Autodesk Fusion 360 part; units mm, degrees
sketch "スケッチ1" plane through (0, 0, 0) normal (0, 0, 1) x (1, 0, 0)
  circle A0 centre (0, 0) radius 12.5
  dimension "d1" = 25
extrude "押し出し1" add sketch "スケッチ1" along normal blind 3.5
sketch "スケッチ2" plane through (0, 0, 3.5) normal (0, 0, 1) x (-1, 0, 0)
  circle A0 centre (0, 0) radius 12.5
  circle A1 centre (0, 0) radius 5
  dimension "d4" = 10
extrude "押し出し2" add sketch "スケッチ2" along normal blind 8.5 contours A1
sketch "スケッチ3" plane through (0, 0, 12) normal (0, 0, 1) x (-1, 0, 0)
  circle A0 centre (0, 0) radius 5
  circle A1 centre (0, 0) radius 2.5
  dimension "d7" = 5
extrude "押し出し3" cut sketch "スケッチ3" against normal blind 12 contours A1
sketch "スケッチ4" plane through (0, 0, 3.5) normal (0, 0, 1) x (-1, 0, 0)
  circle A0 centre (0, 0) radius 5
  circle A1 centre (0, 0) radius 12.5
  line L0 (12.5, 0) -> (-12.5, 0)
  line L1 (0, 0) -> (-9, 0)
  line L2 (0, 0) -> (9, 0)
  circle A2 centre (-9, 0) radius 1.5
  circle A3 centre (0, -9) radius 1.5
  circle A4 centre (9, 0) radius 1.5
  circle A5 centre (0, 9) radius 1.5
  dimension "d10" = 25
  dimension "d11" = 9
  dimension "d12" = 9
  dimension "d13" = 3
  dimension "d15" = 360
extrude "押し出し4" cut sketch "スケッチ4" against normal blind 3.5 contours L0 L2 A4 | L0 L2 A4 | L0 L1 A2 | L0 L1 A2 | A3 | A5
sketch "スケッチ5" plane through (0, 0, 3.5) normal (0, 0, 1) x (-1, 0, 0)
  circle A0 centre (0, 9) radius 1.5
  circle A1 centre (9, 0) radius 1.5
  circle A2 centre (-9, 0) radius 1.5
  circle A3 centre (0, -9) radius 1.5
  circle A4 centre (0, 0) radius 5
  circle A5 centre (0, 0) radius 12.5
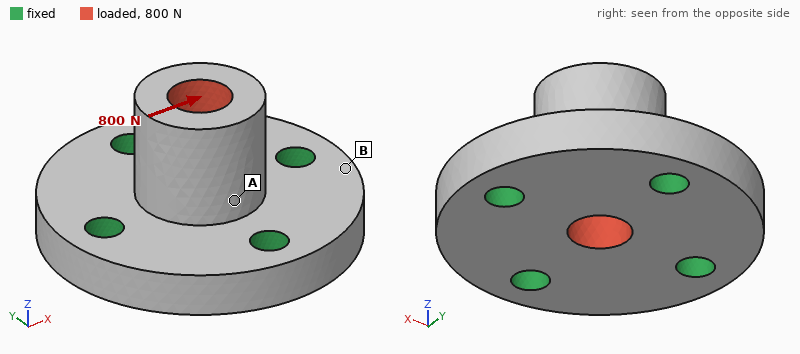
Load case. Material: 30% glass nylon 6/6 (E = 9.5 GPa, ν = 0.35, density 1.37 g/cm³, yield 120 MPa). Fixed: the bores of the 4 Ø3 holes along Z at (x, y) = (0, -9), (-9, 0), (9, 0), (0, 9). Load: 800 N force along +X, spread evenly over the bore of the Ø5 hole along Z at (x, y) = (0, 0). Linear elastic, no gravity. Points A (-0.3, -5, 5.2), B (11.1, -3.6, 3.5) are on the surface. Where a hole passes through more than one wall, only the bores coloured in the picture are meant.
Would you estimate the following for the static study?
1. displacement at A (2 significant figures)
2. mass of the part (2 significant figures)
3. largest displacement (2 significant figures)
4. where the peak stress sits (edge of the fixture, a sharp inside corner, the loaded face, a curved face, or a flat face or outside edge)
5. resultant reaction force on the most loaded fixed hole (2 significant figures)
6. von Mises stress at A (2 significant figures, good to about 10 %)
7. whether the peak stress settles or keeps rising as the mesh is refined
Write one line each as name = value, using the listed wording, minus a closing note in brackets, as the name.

displacement at A = 19 µm
mass of the part = 2.8 g
largest displacement = 64 µm
where the peak stress sits = edge of the fixture
resultant reaction force on the most loaded fixed hole = 350 N
von Mises stress at A = 14 MPa
whether the peak stress settles or keeps rising as the mesh is refined = keeps rising
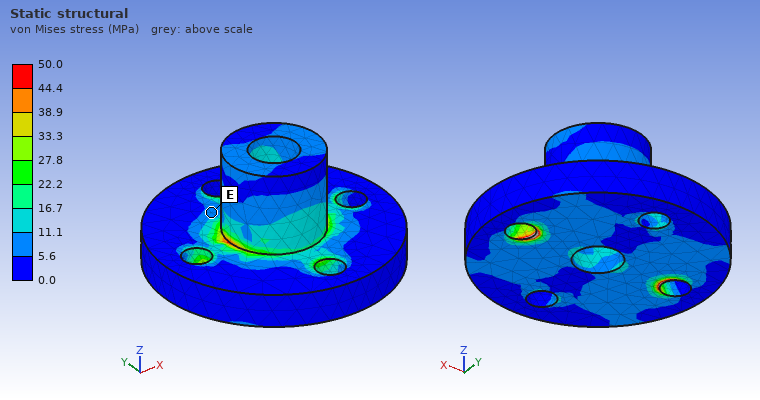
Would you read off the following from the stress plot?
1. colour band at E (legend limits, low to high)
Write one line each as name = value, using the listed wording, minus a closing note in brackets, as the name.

colour band at E = 5.6 to 11.1 MPa
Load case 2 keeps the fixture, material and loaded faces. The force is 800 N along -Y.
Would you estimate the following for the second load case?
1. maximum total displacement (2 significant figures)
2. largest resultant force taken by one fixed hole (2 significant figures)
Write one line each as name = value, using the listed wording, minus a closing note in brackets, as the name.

maximum total displacement = 64 µm
largest resultant force taken by one fixed hole = 350 N
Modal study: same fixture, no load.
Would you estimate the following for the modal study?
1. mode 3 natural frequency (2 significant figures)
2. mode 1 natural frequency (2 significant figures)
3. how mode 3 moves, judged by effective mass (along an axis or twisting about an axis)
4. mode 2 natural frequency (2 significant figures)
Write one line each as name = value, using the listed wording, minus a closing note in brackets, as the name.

mode 3 natural frequency = 30 kHz
mode 1 natural frequency = 21 kHz
how mode 3 moves, judged by effective mass = along Z
mode 2 natural frequency = 21 kHz
